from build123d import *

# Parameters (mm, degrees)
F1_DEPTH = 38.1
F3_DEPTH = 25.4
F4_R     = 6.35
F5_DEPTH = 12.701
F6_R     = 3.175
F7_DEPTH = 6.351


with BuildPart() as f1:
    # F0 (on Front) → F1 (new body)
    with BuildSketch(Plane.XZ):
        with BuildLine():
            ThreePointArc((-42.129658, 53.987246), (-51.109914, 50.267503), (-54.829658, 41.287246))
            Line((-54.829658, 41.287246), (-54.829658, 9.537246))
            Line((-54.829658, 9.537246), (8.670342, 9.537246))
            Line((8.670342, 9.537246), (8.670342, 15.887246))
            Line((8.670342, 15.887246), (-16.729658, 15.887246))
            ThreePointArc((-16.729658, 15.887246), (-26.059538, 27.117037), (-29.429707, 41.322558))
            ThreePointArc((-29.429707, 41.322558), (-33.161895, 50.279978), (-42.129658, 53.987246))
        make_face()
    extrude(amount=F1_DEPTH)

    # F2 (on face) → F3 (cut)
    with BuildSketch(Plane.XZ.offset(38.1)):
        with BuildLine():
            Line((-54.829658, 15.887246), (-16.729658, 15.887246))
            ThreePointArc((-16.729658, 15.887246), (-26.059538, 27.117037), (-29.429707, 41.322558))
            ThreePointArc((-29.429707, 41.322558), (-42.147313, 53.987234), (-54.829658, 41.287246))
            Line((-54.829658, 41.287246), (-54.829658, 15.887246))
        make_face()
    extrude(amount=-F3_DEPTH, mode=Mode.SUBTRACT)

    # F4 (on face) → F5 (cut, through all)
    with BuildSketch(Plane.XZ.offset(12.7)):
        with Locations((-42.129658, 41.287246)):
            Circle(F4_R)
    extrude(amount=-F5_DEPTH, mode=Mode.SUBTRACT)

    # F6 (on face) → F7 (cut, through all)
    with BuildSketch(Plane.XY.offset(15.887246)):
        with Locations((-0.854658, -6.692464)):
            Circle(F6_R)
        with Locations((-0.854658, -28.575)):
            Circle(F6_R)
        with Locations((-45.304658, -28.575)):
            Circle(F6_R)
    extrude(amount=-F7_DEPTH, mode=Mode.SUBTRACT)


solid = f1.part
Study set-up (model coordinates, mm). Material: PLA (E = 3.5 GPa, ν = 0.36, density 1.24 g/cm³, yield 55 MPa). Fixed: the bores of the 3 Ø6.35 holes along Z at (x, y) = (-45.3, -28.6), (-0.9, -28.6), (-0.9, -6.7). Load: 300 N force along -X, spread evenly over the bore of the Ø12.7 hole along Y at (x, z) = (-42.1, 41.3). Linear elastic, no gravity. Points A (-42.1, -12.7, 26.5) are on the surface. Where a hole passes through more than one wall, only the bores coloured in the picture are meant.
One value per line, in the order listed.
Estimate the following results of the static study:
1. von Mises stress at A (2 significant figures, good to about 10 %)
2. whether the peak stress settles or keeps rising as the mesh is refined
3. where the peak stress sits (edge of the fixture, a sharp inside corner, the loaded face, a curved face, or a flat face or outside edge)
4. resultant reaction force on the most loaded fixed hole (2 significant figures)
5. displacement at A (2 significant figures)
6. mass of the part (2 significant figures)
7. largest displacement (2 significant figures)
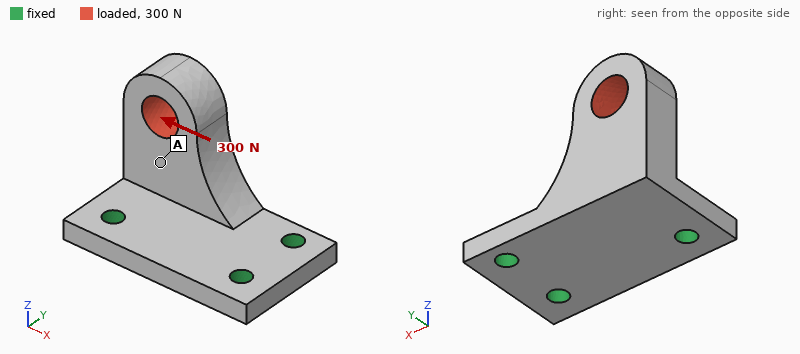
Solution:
3.5 MPa
keeps rising
edge of the fixture
230 N
0.20 mm
32 g
0.56 mm
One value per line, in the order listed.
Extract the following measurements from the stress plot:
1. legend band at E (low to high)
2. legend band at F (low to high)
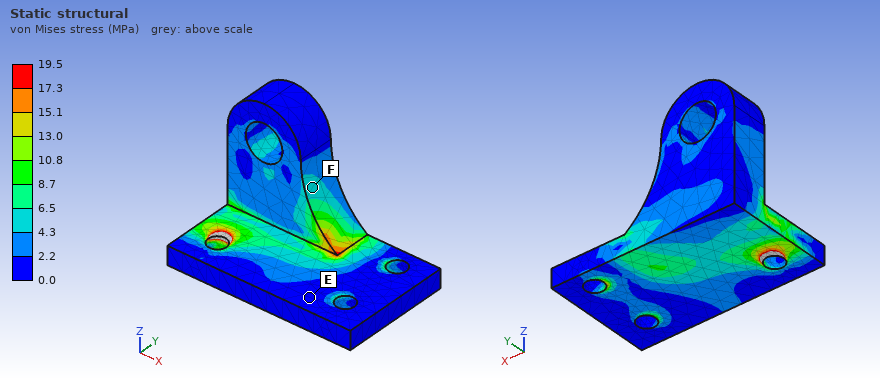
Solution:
0.0 to 2.2 MPa
4.3 to 6.5 MPa
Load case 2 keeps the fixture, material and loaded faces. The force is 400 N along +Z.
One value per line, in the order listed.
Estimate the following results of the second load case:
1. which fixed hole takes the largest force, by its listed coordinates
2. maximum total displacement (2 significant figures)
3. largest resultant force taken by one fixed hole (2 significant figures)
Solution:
(-45.3, -28.6)
0.87 mm
330 N
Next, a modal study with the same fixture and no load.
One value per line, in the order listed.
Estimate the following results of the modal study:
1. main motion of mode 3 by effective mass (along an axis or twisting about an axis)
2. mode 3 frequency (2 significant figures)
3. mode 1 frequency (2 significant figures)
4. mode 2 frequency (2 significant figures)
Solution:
along Z
2800 Hz
840 Hz
1900 Hz
